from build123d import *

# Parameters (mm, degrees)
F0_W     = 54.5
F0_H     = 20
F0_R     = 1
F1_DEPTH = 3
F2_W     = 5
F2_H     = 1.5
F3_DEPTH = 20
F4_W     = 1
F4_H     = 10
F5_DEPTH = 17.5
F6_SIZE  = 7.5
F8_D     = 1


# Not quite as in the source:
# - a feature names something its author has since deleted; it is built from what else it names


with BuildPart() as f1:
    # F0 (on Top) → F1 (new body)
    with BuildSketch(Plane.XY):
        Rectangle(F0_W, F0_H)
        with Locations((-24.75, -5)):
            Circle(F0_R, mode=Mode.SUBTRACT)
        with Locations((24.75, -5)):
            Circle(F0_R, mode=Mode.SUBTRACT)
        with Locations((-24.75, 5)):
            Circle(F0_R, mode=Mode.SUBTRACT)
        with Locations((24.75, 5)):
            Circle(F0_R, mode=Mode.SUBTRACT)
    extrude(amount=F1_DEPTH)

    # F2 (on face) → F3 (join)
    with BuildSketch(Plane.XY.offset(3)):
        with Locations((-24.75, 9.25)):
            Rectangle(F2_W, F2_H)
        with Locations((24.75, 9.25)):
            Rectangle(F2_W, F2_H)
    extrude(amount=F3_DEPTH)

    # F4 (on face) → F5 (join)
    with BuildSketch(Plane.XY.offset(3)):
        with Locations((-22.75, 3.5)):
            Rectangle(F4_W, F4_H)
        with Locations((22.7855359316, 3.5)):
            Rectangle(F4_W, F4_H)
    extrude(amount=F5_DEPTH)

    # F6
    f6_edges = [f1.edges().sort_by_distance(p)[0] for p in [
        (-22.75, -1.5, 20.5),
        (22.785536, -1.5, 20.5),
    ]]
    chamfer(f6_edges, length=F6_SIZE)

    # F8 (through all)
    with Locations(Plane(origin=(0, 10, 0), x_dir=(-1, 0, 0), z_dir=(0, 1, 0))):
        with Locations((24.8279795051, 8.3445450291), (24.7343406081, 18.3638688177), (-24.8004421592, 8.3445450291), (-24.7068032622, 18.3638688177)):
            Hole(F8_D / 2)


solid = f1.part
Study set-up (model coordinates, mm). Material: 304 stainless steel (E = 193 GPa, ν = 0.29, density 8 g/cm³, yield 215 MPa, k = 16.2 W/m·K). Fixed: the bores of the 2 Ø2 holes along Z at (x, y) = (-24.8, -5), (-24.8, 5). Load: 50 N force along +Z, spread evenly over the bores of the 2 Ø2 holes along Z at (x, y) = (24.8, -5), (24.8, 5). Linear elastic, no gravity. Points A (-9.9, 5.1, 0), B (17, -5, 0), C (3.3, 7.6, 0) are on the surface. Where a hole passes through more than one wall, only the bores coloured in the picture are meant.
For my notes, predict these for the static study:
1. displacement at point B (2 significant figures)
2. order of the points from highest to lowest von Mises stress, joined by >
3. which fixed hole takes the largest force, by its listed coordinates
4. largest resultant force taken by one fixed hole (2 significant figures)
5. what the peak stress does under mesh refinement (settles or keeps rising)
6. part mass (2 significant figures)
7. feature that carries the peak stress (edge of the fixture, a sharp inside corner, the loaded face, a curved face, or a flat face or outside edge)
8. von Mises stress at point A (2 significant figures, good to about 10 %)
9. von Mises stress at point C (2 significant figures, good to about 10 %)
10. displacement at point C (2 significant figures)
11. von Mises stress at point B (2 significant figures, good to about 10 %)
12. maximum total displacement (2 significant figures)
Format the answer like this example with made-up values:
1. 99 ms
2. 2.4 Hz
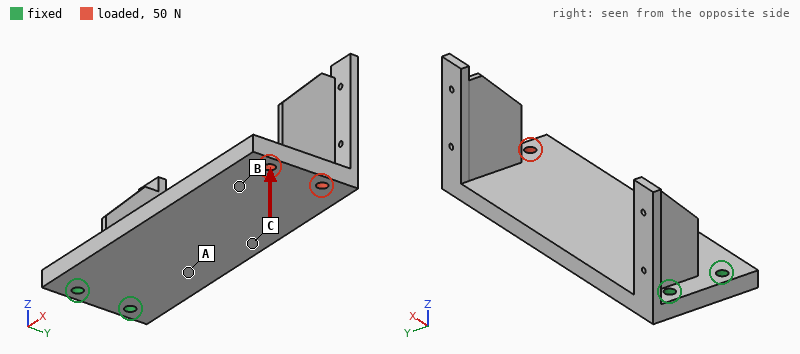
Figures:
1. 0.18 mm
2. A > C > B
3. (-24.8, -5)
4. 28 N
5. keeps rising
6. 31 g
7. edge of the fixture
8. 56 MPa
9. 36 MPa
10. 0.092 mm
11. 14 MPa
12. 0.29 mm
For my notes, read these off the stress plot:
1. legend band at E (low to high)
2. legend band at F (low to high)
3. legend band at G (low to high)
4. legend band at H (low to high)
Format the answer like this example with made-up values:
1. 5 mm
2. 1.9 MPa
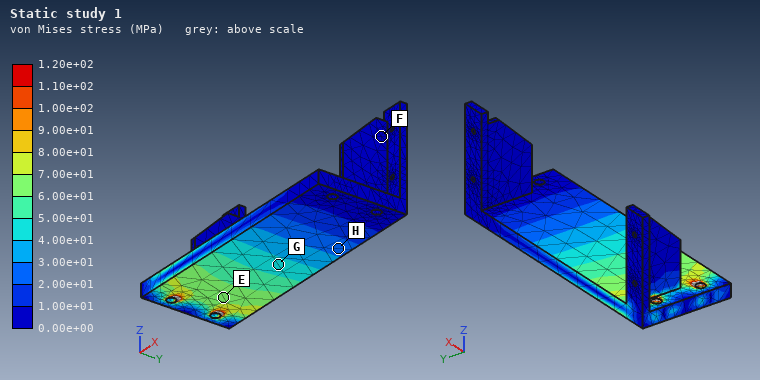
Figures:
1. 6.00e+01 to 7.00e+01 MPa
2. 0.00e+00 to 1.00e+01 MPa
3. 4.00e+01 to 5.00e+01 MPa
4. 2.00e+01 to 3.00e+01 MPa
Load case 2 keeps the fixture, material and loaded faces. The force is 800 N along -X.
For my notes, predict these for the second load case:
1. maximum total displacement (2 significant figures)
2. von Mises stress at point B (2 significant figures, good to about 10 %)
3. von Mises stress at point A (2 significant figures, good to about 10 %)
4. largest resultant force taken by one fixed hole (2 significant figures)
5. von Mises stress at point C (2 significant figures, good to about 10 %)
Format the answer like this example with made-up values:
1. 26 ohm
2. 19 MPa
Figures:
1. 4.1 µm
2. 14 MPa
3. 13 MPa
4. 400 N
5. 13 MPa
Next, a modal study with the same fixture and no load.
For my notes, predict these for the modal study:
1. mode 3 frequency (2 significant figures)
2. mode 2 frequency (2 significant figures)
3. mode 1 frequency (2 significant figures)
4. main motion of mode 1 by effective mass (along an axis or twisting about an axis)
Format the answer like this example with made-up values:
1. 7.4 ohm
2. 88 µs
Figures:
1. 3800 Hz
2. 2900 Hz
3. 760 Hz
4. along Z
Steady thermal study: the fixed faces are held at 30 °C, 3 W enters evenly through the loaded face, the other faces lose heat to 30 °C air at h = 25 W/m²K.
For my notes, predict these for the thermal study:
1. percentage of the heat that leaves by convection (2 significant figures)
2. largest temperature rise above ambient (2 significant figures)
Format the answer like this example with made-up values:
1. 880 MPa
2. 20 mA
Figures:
1. 76 %
2. 70 K
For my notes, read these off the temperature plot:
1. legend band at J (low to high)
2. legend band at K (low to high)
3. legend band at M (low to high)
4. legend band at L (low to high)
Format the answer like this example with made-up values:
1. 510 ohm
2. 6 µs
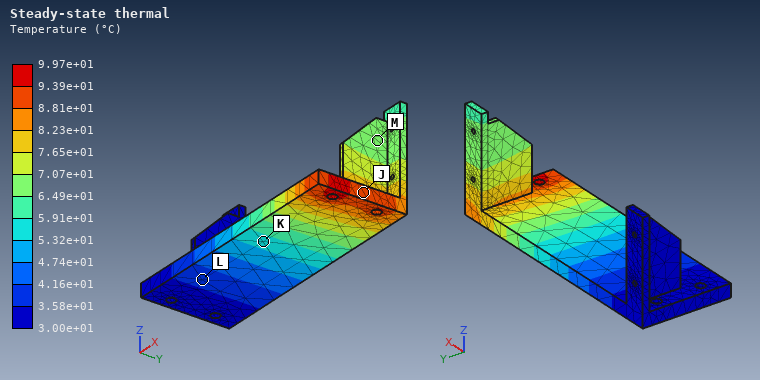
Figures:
1. 8.81e+01 to 9.39e+01 °C
2. 5.32e+01 to 5.91e+01 °C
3. 6.49e+01 to 7.07e+01 °C
4. 3.58e+01 to 4.16e+01 °C
